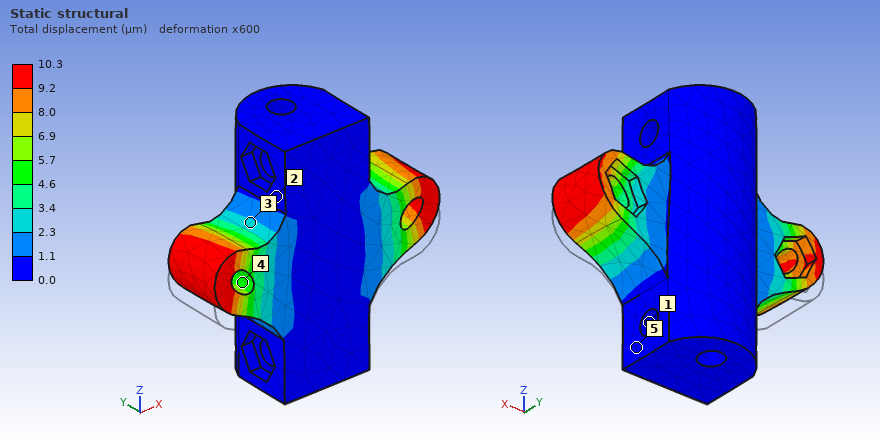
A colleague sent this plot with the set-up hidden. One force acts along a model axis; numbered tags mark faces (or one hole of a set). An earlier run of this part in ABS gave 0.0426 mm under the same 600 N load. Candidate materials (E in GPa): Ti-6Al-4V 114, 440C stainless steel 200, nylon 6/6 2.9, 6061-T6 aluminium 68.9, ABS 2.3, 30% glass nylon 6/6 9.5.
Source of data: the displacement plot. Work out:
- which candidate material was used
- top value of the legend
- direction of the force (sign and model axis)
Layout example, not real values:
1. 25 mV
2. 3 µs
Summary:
1. 30% glass nylon 6/6
2. 10.3 µm
3. +Z
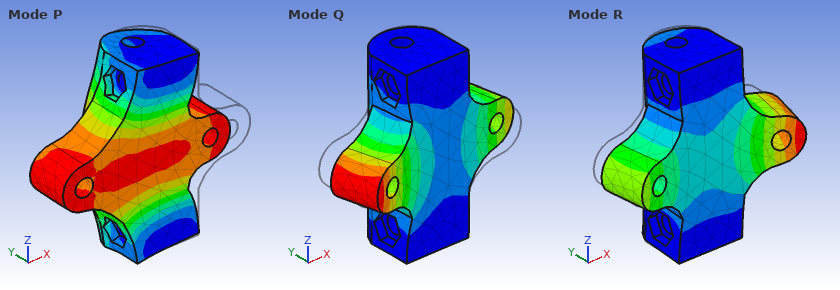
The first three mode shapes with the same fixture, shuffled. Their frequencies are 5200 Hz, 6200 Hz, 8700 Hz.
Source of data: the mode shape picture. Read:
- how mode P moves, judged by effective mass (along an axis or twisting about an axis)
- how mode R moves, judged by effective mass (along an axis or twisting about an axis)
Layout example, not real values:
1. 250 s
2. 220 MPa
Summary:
1. along X
2. along Y
